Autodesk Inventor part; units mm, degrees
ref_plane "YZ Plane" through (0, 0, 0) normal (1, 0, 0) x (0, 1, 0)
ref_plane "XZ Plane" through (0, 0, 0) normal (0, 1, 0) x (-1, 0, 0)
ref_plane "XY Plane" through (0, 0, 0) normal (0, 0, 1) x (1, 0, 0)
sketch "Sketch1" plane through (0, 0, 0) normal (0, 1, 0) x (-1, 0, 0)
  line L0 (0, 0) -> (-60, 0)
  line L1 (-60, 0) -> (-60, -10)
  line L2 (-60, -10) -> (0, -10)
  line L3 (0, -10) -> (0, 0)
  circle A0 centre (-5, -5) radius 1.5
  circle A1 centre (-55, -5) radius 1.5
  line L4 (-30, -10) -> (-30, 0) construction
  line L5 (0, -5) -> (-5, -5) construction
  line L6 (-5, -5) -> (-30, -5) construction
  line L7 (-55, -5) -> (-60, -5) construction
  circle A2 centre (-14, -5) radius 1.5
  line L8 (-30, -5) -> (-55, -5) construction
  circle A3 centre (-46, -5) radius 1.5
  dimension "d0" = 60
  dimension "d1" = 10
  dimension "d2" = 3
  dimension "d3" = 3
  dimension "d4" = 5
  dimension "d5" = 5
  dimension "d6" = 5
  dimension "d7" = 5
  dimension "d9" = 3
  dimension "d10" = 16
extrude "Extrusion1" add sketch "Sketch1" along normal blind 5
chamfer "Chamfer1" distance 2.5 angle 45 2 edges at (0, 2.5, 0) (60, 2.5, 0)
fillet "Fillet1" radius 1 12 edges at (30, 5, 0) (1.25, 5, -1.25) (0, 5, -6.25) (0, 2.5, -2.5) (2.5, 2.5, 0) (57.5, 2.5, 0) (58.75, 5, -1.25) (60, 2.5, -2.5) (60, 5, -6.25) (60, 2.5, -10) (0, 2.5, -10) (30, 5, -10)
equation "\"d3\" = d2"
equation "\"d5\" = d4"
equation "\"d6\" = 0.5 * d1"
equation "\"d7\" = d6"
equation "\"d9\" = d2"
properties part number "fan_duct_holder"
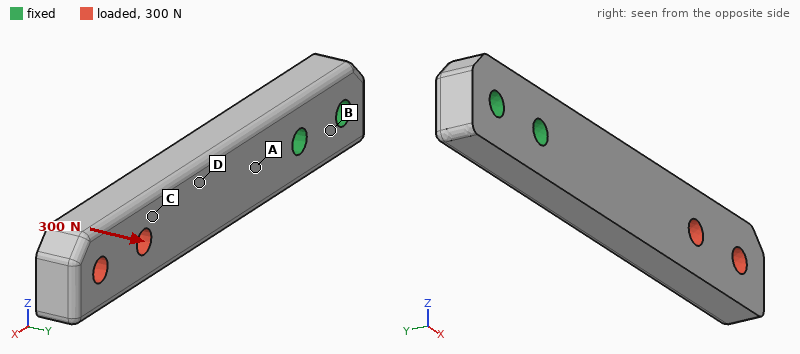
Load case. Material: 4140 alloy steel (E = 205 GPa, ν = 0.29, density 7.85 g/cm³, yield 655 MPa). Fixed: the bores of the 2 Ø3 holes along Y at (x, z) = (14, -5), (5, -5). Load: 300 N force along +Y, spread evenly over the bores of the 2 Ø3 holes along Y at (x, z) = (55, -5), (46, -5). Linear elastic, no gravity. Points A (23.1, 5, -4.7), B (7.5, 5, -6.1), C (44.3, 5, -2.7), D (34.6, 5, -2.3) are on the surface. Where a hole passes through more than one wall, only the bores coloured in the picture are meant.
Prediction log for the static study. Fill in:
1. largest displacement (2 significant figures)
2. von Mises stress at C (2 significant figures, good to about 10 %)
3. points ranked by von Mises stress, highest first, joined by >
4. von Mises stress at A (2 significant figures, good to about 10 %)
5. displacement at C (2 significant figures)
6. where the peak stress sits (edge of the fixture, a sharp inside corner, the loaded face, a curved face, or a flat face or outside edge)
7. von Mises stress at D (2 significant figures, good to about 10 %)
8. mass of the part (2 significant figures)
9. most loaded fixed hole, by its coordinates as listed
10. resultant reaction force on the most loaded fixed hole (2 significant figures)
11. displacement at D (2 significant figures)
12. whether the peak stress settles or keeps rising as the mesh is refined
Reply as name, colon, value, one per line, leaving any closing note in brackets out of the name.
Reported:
largest displacement: 0.32 mm
von Mises stress at C: 62 MPa
points ranked by von Mises stress, highest first, joined by >: A > D > C > B
von Mises stress at A: 200 MPa
displacement at C: 0.17 mm
where the peak stress sits: edge of the fixture
von Mises stress at D: 120 MPa
mass of the part: 22 g
most loaded fixed hole, by its coordinates as listed: (14, -5)
resultant reaction force on the most loaded fixed hole: 530 N
displacement at D: 0.091 mm
whether the peak stress settles or keeps rising as the mesh is refined: keeps rising
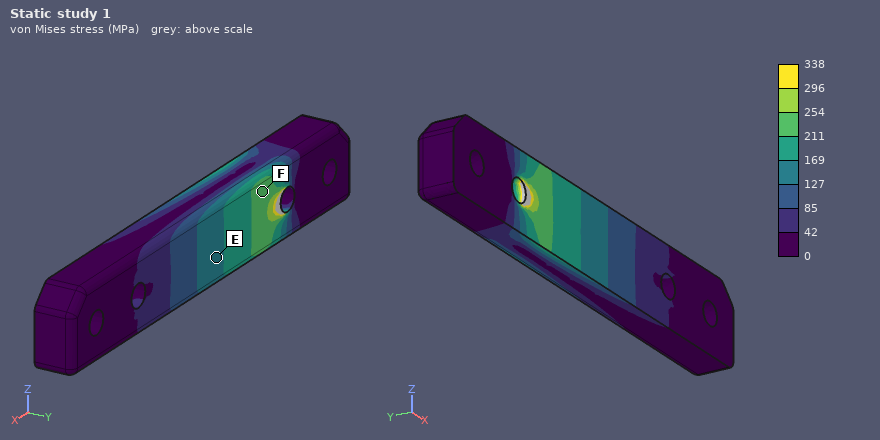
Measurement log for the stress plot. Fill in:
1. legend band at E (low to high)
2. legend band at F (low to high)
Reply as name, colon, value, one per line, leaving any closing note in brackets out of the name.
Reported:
legend band at E: 127 to 169 MPa
legend band at F: 211 to 254 MPa
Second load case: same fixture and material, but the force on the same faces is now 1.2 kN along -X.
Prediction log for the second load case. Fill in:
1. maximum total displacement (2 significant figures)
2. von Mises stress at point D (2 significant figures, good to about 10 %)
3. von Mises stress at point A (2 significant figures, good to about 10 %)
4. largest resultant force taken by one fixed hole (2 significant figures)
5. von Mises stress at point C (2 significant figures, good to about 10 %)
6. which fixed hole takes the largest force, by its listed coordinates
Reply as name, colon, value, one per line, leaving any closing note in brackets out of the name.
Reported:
maximum total displacement: 5.1 µm
von Mises stress at point D: 25 MPa
von Mises stress at point A: 26 MPa
largest resultant force taken by one fixed hole: 1.1 kN
von Mises stress at point C: 33 MPa
which fixed hole takes the largest force, by its listed coordinates: (14, -5)
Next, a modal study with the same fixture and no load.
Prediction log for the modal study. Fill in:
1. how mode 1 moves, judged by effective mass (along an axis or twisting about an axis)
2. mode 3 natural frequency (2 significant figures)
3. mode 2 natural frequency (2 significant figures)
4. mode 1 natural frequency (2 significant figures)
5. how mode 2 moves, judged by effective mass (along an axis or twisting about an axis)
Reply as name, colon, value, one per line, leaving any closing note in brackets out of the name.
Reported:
how mode 1 moves, judged by effective mass: along Y
mode 3 natural frequency: 12 kHz
mode 2 natural frequency: 3500 Hz
mode 1 natural frequency: 2000 Hz
how mode 2 moves, judged by effective mass: along Z
